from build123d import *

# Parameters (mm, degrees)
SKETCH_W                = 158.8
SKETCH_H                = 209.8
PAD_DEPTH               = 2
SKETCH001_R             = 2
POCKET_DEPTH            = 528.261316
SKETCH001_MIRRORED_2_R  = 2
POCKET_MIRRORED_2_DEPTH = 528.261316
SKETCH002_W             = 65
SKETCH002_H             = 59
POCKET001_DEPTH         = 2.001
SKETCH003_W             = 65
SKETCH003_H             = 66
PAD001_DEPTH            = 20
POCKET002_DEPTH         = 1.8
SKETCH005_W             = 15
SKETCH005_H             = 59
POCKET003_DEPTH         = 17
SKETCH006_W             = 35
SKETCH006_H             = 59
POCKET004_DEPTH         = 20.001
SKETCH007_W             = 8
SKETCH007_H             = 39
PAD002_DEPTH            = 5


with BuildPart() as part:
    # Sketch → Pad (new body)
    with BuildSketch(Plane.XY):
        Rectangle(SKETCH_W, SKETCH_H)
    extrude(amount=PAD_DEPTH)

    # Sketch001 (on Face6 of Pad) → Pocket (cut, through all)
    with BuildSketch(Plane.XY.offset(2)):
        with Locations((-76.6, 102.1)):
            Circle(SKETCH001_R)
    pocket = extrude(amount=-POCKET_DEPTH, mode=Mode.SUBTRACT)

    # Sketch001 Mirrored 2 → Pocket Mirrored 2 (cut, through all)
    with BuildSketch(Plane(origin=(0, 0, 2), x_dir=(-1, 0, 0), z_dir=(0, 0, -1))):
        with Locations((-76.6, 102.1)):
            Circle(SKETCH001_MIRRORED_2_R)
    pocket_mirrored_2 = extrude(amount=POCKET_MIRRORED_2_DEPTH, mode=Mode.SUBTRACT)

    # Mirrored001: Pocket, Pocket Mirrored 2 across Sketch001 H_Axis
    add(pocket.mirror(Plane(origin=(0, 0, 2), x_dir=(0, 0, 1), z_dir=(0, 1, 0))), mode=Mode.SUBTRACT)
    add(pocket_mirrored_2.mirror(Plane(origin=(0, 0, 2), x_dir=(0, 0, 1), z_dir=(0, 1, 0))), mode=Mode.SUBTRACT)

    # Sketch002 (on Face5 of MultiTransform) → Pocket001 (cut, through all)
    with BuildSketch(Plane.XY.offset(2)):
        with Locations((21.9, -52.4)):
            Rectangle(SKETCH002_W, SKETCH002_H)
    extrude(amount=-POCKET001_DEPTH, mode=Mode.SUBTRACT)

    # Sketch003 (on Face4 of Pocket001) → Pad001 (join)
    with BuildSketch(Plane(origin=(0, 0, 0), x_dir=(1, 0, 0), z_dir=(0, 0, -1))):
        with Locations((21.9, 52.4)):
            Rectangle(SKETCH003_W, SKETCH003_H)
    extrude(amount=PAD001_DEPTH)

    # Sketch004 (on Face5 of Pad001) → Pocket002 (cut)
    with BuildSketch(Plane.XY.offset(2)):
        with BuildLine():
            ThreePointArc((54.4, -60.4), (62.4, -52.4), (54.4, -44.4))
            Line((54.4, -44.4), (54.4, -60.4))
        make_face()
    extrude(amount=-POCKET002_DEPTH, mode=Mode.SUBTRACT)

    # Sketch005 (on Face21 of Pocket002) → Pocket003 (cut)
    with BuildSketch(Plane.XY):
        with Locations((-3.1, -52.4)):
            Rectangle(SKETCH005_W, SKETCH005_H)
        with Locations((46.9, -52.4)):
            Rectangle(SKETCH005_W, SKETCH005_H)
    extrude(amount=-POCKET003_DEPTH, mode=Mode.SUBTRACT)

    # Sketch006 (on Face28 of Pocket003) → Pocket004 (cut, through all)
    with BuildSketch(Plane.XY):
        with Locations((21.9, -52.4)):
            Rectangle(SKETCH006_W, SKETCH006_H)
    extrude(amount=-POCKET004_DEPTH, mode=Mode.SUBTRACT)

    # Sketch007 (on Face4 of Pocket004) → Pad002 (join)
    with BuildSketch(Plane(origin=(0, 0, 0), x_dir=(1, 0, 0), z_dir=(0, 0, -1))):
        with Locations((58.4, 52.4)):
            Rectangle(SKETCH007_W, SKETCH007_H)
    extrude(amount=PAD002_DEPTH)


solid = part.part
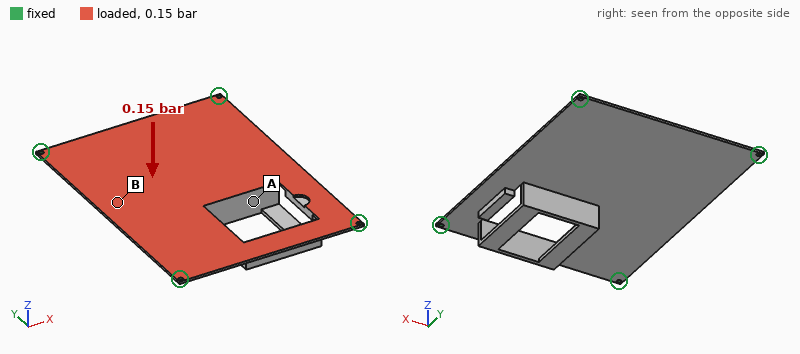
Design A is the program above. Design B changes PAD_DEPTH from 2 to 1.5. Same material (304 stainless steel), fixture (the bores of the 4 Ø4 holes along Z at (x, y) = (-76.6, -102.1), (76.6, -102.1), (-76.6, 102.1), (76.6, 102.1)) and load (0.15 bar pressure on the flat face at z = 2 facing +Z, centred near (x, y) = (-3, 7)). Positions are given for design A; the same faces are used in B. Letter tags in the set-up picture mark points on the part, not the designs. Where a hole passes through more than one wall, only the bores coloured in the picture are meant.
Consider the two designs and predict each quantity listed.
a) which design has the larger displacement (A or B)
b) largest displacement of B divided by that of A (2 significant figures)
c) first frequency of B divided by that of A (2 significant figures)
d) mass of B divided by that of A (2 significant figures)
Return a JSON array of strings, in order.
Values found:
["B", "2.3", "0.74", "0.80"]
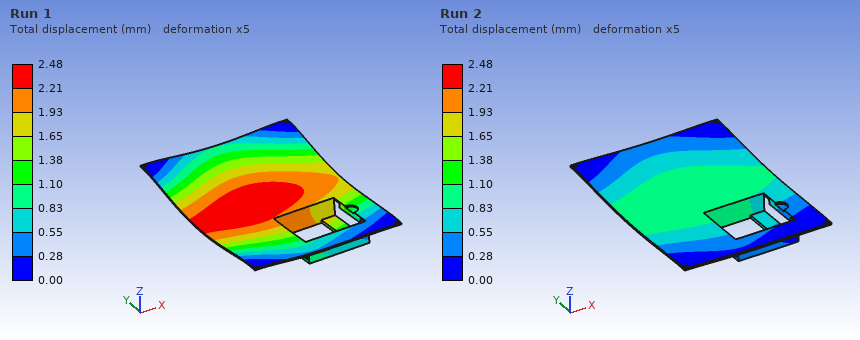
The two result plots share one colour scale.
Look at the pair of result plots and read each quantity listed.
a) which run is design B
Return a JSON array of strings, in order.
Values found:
["Run 1"]
